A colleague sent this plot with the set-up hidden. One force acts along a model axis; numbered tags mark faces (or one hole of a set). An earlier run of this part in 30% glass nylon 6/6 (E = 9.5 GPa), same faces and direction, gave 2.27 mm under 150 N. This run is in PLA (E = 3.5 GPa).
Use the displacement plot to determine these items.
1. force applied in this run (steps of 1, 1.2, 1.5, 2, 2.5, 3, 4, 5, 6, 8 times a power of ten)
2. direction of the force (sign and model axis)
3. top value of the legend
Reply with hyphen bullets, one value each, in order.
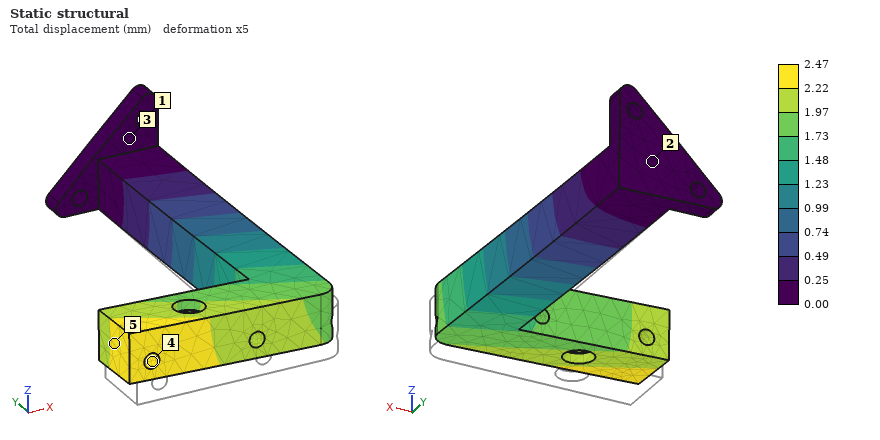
- 60 N
- +Z
- 2.47 mm
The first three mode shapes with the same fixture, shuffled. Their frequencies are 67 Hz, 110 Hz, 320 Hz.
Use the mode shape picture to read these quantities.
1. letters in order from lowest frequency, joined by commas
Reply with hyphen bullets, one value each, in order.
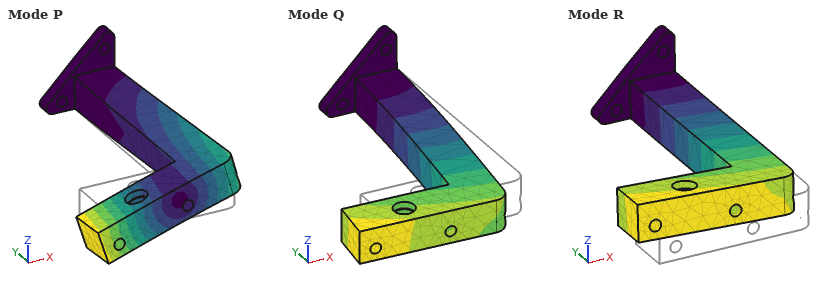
- R, Q, P
